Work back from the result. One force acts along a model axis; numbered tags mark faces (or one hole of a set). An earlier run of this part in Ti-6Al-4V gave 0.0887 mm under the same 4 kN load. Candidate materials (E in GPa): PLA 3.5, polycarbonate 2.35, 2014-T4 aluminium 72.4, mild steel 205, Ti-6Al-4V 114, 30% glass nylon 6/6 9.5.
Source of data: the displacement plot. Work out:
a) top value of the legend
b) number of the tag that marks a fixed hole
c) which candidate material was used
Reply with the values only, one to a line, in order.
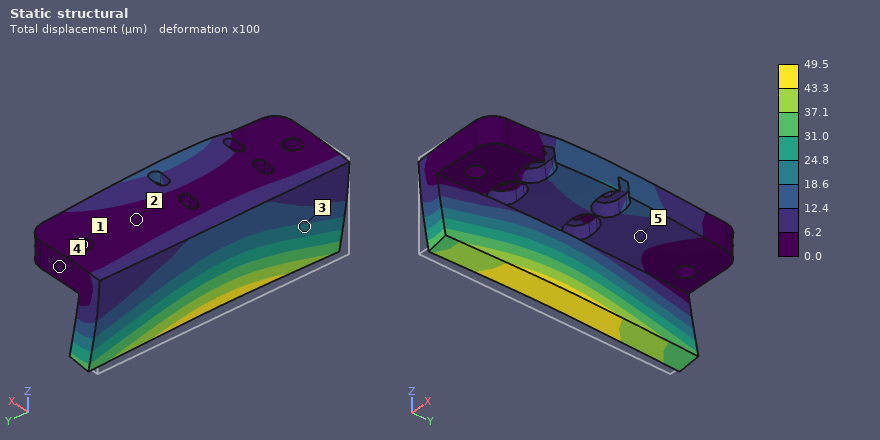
49.5 µm
1
mild steel
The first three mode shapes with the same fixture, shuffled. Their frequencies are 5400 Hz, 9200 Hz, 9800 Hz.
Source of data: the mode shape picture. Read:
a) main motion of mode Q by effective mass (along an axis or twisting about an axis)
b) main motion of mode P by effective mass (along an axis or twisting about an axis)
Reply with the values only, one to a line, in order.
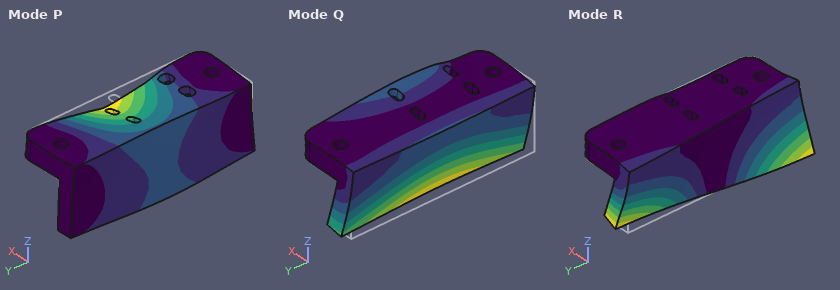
along X
along Z
